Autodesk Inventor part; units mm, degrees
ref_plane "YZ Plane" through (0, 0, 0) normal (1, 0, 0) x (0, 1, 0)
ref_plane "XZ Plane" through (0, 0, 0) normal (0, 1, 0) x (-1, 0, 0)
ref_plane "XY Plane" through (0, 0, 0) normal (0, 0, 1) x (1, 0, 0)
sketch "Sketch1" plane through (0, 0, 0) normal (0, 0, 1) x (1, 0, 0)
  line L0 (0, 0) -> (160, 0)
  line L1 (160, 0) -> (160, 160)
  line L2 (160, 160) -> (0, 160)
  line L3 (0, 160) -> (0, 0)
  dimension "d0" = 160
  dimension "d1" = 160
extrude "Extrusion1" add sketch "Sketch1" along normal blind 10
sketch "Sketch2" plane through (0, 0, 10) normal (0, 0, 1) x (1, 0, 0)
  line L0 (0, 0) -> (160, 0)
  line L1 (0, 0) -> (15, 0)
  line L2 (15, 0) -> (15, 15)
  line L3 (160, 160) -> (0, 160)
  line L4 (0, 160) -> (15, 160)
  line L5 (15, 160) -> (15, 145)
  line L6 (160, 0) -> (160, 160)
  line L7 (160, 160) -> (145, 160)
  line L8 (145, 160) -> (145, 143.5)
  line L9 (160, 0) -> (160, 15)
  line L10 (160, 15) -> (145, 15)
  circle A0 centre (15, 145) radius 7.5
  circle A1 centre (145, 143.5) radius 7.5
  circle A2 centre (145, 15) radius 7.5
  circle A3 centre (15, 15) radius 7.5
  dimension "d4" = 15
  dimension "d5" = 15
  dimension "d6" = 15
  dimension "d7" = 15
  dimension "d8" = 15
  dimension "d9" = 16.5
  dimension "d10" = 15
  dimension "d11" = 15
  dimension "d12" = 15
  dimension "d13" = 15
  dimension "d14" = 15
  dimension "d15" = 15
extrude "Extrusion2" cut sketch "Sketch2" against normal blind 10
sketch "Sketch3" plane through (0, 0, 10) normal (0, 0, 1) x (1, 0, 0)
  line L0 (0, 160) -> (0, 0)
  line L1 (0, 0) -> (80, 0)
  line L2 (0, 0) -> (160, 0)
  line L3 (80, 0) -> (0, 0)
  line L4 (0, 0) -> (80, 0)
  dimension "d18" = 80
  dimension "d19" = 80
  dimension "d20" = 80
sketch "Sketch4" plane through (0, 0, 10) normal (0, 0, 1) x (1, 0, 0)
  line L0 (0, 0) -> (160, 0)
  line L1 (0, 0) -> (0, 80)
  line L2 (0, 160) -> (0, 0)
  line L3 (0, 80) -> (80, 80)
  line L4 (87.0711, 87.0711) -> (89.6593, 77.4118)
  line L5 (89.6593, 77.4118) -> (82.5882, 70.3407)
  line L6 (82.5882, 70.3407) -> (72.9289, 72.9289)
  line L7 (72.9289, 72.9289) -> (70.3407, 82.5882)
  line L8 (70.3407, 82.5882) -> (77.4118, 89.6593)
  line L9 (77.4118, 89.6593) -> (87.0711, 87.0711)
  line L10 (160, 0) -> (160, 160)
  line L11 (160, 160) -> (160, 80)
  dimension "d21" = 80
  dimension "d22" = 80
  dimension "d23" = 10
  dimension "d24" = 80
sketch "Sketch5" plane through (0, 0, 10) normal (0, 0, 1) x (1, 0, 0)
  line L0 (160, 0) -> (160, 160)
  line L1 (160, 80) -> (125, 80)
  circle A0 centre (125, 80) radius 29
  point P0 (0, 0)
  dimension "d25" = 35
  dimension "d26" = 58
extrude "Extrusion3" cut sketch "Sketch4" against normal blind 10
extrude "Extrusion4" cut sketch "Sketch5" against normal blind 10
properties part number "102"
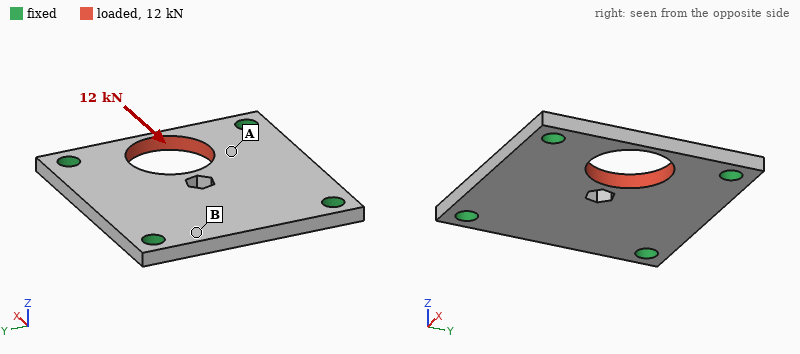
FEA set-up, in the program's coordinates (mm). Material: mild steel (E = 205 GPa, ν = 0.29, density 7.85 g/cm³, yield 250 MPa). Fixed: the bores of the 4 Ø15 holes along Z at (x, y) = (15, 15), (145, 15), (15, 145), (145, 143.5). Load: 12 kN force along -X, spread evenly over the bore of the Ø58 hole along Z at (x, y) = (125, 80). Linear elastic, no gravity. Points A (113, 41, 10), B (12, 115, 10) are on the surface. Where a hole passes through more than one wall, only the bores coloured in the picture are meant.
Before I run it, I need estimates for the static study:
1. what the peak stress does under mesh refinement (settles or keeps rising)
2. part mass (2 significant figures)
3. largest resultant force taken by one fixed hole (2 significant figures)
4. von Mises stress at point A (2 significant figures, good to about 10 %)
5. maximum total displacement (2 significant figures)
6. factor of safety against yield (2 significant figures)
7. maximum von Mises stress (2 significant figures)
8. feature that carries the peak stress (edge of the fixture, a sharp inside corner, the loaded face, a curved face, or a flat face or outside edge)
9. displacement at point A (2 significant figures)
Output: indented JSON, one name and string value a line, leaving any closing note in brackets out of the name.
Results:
{
  "what the peak stress does under mesh refinement": "settles",
  "part mass": "1.7 kg",
  "largest resultant force taken by one fixed hole": "3.6 kN",
  "von Mises stress at point A": "13 MPa",
  "maximum total displacement": "17 µm",
  "factor of safety against yield": "3.7",
  "maximum von Mises stress": "68 MPa",
  "feature that carries the peak stress": "a flat face or outside edge",
  "displacement at point A": "2.9 µm"
}
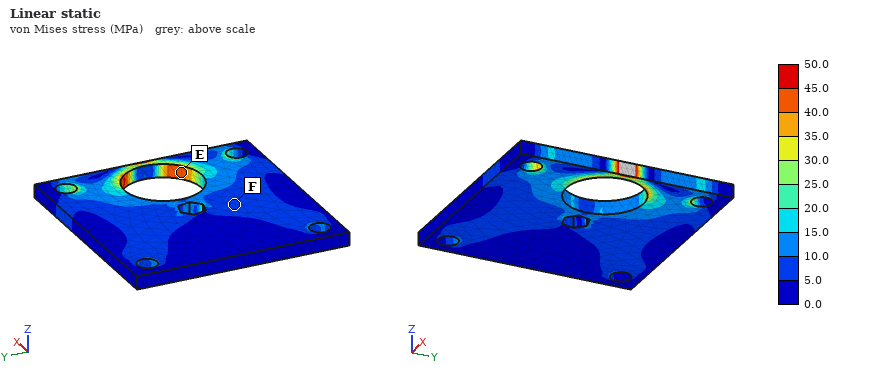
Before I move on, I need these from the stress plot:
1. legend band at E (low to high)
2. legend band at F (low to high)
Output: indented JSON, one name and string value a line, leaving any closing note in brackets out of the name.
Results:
{
  "legend band at E": "40.0 to 45.0 MPa",
  "legend band at F": "5.0 to 10.0 MPa"
}
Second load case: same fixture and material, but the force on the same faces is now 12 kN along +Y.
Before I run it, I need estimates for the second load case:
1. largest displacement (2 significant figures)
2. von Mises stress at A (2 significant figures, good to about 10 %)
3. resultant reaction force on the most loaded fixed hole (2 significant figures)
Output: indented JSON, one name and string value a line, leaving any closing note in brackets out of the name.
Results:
{
  "largest displacement": "3.5 µm",
  "von Mises stress at A": "6.6 MPa",
  "resultant reaction force on the most loaded fixed hole": "4.6 kN"
}
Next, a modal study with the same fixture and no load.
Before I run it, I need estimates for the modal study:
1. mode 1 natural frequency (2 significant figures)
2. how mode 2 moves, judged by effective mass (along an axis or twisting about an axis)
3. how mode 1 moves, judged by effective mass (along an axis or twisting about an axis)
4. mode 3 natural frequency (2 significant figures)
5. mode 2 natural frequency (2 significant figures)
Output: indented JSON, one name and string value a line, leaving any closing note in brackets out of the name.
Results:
{
  "mode 1 natural frequency": "2300 Hz",
  "how mode 2 moves, judged by effective mass": "twisting about X",
  "how mode 1 moves, judged by effective mass": "along Z",
  "mode 3 natural frequency": "3800 Hz",
  "mode 2 natural frequency": "3600 Hz"
}
